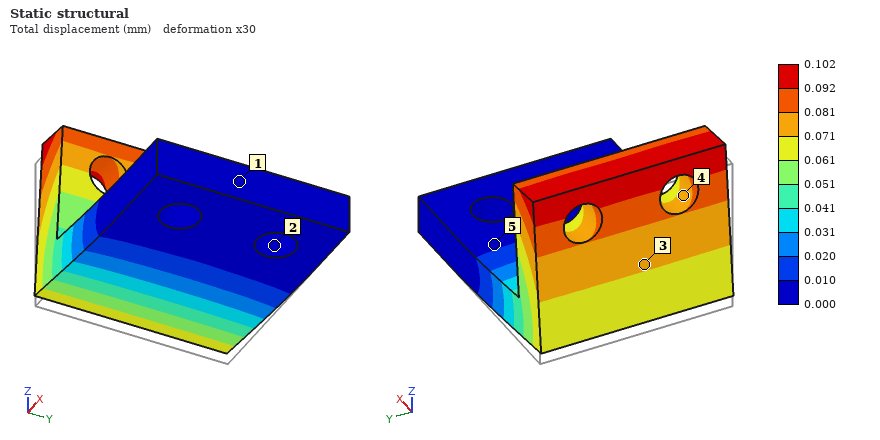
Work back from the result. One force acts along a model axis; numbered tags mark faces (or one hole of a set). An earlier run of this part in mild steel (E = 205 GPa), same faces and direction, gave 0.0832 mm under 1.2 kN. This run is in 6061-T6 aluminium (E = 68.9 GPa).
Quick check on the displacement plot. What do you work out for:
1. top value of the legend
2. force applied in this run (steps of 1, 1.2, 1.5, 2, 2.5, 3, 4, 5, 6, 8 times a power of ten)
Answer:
0.102 mm
500 N
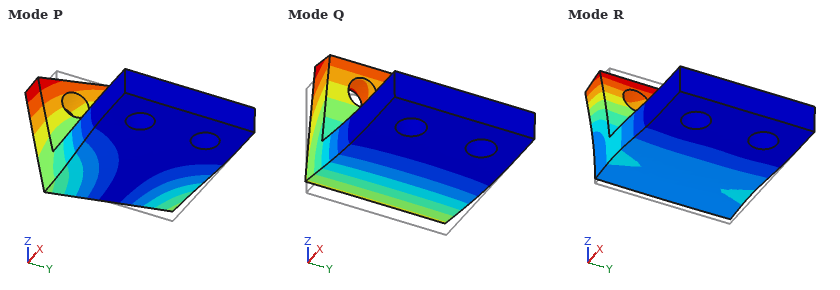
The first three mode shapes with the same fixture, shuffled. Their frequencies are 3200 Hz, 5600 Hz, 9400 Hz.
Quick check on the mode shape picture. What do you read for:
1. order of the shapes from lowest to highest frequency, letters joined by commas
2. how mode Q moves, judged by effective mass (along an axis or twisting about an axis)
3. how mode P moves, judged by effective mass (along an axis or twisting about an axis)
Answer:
Q, P, R
along Z
along Y
